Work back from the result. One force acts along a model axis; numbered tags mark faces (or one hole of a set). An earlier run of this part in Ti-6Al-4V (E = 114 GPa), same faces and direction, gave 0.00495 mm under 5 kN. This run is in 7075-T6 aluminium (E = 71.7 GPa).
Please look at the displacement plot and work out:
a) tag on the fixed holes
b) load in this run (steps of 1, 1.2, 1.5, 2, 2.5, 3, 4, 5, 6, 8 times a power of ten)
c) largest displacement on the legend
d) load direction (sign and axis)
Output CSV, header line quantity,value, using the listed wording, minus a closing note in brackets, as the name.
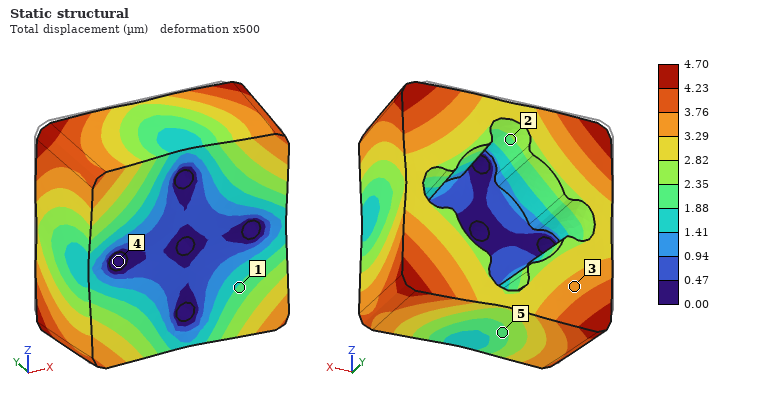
quantity,value
tag on the fixed holes,4
load in this run,3 kN
largest displacement on the legend,4.70 µm
load direction,-Y
